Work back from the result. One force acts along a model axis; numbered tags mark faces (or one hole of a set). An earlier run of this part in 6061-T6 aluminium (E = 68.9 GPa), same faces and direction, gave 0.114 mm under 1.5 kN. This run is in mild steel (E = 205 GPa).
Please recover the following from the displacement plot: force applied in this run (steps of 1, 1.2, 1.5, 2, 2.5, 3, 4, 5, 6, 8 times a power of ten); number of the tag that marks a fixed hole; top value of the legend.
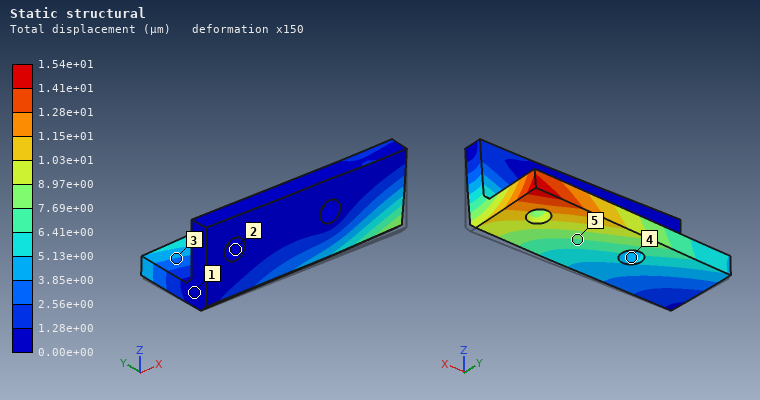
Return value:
600 N
2
1.54e+01 µm
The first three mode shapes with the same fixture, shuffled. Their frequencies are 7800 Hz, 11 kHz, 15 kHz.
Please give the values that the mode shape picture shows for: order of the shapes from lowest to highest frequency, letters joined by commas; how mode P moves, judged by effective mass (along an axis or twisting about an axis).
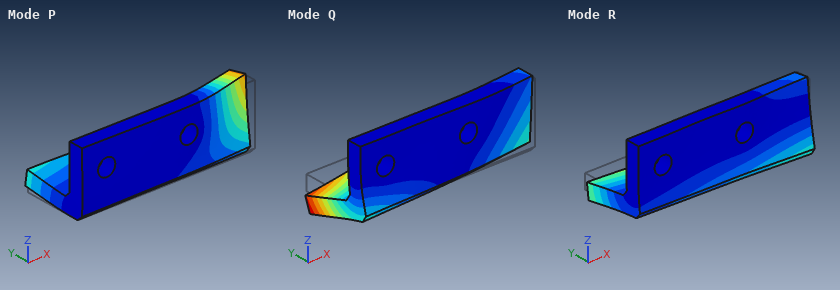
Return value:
R, Q, P
along Y
